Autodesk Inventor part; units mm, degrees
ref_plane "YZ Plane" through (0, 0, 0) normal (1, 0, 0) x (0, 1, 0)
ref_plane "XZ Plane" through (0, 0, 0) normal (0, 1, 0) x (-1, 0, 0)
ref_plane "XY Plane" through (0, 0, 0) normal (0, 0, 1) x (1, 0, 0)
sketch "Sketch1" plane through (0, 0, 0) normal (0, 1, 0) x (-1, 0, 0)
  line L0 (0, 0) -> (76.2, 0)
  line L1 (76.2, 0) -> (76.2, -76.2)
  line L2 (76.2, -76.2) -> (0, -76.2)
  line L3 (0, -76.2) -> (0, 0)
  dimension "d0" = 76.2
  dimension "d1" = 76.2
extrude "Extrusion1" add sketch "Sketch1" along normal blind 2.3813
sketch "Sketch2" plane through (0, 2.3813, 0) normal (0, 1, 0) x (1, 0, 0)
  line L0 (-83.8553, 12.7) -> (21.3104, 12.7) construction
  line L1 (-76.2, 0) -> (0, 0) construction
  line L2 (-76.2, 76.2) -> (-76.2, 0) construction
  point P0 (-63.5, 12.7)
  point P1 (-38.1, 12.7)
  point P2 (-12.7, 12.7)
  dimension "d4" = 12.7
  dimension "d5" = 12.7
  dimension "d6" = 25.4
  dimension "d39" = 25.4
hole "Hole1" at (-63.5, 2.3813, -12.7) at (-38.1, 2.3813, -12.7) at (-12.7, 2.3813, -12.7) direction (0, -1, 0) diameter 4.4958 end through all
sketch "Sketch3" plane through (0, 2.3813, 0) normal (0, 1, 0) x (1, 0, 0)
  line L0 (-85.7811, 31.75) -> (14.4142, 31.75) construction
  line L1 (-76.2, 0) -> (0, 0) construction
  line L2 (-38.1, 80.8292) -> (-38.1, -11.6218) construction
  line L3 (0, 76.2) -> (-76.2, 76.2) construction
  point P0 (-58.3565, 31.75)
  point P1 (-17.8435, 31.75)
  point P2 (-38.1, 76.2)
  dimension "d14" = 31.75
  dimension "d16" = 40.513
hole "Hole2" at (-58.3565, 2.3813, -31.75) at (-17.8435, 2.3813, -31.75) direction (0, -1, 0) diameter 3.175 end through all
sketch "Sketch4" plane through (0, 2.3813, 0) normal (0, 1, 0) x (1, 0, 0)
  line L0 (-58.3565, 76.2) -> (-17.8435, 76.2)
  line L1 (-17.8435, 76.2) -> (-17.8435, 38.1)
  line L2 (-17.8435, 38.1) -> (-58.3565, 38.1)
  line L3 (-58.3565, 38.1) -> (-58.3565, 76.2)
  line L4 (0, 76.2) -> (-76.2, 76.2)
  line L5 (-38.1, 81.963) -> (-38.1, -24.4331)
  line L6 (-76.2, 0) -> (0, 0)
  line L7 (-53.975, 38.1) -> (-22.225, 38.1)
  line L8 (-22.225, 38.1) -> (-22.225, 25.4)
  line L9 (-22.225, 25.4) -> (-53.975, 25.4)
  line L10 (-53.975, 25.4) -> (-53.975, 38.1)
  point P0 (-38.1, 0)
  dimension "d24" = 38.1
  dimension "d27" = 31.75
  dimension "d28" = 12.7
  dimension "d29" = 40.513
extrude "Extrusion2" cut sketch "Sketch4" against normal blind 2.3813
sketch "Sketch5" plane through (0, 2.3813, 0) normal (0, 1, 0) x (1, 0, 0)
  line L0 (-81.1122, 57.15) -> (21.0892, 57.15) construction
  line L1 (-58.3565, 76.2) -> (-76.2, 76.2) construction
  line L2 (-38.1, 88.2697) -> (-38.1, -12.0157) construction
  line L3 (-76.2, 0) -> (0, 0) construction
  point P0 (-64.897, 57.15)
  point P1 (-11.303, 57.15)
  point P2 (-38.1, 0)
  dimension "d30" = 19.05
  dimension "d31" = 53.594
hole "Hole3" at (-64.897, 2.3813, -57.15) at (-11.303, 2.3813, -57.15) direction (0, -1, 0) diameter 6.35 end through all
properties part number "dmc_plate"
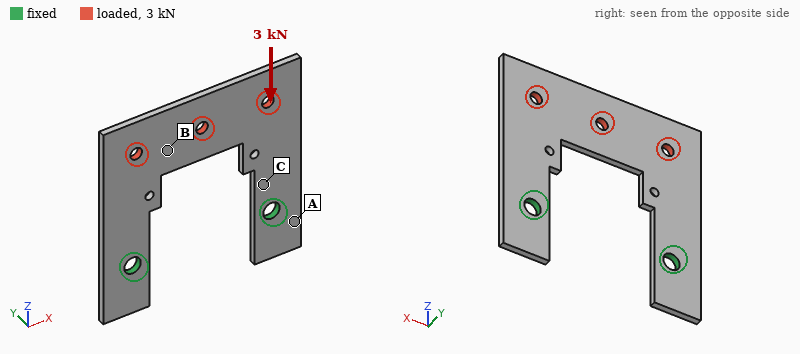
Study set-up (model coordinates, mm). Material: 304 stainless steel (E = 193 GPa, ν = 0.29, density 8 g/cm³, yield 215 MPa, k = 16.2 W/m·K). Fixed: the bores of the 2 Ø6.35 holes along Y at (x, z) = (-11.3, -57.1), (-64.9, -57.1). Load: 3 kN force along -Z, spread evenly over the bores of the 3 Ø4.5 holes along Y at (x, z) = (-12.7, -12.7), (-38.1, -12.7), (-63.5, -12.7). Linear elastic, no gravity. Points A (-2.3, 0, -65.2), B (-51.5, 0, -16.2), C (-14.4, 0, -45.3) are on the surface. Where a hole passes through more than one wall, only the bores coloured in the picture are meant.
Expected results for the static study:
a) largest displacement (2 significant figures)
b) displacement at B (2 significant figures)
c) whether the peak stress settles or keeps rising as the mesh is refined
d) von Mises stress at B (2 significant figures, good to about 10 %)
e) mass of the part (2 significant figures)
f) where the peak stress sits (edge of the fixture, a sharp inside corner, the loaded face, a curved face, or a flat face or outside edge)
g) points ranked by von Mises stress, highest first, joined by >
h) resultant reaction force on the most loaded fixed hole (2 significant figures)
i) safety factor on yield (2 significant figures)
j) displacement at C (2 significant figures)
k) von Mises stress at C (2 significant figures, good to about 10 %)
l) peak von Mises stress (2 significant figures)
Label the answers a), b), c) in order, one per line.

a) 14 µm
b) 11 µm
c) settles
d) 22 MPa
e) 71 g
f) a curved face
g) C > B > A
h) 1.5 kN
i) 1.5
j) 2.8 µm
k) 50 MPa
l) 140 MPa
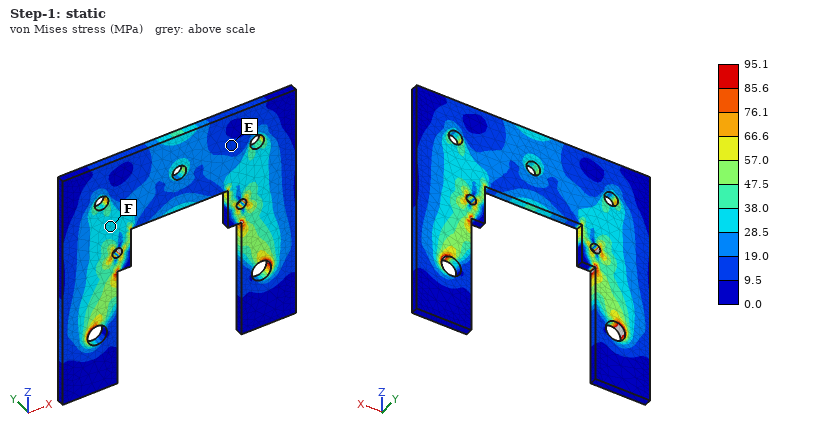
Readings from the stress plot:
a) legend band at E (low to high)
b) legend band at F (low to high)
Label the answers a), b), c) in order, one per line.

a) 9.5 to 19.0 MPa
b) 28.5 to 38.0 MPa
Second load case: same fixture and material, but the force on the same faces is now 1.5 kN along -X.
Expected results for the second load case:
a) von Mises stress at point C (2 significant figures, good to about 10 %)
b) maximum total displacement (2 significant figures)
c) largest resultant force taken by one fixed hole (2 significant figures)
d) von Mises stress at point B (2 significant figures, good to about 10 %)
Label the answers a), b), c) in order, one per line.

a) 36 MPa
b) 41 µm
c) 1.1 kN
d) 36 MPa
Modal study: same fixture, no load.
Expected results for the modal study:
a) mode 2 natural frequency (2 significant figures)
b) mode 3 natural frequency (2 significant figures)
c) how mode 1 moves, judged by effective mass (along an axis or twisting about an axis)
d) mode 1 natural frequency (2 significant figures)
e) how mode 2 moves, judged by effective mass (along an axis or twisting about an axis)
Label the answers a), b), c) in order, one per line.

a) 1000 Hz
b) 2500 Hz
c) along Y
d) 440 Hz
e) twisting about Z
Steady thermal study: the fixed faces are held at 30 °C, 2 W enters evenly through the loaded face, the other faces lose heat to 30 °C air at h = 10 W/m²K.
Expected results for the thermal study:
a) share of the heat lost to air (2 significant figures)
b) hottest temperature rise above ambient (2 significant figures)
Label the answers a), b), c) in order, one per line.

a) 62 %
b) 29 K
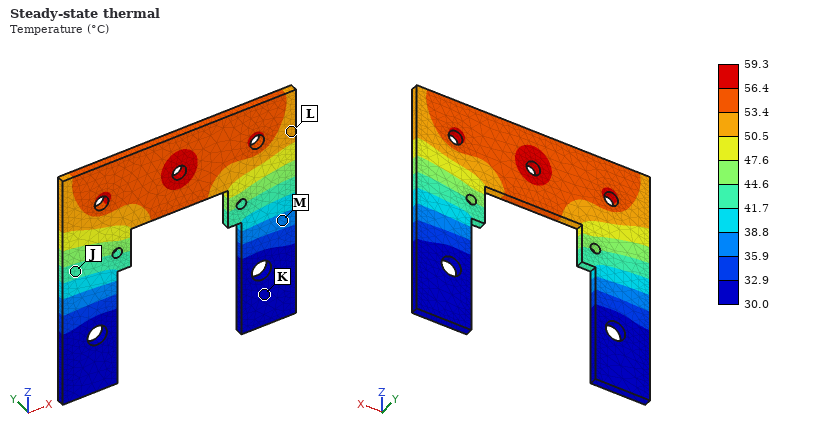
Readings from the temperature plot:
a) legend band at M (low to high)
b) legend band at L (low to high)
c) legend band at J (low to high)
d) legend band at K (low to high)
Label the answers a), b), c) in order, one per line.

a) 35.9 to 38.8 °C
b) 50.5 to 53.4 °C
c) 41.7 to 44.6 °C
d) 30.0 to 32.9 °C
